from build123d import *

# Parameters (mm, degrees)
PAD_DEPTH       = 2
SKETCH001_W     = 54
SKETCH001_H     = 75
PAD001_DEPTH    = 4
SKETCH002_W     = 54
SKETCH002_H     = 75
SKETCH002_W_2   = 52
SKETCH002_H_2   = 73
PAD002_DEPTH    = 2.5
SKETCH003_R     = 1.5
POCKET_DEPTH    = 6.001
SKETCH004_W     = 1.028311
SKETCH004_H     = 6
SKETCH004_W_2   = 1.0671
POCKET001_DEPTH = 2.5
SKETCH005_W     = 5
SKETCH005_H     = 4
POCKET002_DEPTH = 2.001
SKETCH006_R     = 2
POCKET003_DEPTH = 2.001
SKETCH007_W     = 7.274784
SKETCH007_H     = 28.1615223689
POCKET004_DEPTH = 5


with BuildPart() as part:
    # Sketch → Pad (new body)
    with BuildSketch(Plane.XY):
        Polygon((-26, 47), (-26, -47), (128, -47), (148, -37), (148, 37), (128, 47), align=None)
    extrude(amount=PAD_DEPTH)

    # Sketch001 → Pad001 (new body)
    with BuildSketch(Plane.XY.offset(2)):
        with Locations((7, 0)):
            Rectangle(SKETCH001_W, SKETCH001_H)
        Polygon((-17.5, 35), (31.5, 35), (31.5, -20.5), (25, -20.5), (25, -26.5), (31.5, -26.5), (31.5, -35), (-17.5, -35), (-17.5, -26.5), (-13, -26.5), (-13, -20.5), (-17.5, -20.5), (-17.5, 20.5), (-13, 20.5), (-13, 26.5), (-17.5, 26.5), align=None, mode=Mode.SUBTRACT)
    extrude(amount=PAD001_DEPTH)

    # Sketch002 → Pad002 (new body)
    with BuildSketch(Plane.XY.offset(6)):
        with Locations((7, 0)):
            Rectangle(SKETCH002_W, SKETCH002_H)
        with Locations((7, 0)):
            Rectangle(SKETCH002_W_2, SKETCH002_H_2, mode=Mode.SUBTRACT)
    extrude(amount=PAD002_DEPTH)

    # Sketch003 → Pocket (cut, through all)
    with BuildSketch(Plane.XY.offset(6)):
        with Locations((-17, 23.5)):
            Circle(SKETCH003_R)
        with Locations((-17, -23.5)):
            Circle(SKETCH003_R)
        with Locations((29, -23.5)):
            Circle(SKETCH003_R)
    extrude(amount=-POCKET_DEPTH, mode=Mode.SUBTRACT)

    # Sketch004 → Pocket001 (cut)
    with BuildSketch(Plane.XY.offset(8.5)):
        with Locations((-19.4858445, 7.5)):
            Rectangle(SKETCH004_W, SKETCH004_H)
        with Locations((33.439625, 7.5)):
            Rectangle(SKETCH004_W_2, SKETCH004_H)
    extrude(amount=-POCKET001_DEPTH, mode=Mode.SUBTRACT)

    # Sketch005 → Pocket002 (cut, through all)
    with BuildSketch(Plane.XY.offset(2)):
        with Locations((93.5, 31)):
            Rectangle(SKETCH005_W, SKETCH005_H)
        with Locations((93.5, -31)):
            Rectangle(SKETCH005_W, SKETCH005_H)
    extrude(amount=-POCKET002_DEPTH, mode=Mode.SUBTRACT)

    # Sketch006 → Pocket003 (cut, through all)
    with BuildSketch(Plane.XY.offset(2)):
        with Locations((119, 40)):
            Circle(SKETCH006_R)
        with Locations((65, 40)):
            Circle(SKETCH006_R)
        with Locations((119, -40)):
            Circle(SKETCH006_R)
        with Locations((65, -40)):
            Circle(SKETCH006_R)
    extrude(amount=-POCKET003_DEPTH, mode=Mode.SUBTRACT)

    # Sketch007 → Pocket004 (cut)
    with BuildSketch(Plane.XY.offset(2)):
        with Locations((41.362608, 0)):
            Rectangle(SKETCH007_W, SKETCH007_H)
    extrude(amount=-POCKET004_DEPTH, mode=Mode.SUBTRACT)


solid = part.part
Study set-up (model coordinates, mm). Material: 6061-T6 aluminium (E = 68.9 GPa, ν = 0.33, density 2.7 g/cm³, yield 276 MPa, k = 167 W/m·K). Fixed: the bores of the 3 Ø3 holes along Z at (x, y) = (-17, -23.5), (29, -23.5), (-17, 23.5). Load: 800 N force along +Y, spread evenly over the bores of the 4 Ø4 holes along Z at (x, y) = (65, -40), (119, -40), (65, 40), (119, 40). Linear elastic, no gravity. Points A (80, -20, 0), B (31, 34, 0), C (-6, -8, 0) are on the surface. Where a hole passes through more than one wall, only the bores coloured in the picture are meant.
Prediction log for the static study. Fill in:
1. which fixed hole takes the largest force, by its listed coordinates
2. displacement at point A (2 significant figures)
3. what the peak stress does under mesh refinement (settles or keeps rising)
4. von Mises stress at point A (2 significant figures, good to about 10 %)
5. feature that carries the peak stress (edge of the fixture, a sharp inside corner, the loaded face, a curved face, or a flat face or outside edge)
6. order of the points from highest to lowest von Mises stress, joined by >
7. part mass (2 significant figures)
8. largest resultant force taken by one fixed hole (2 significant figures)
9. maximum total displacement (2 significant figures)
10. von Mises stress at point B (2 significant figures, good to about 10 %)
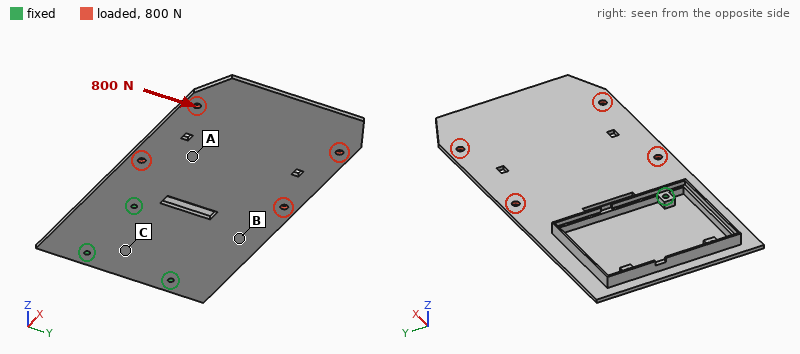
(29, -23.5)
36 µm
keeps rising
6.1 MPa
edge of the fixture
B > A > C
95 g
1.2 kN
80 µm
13 MPa
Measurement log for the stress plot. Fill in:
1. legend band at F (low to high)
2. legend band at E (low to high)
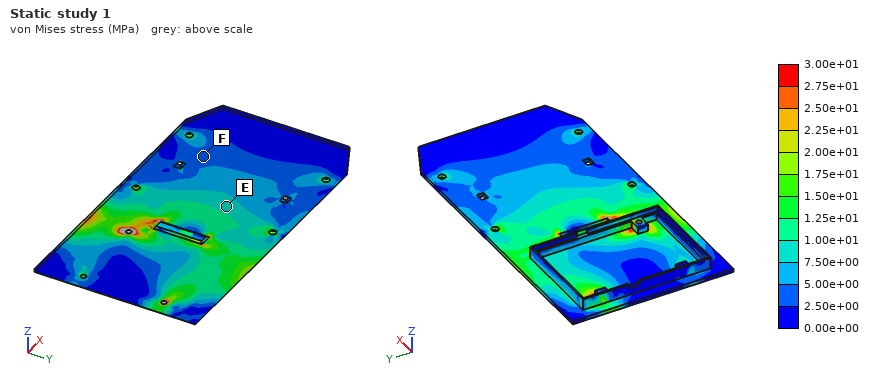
2.50e+00 to 5.00e+00 MPa
7.50e+00 to 1.00e+01 MPa
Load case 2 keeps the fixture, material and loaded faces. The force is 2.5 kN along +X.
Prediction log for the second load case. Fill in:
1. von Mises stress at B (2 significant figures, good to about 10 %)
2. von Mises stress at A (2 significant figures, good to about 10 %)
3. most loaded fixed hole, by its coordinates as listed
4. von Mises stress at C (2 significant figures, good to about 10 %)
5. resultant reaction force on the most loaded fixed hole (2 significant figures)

18 MPa
9.0 MPa
(29, -23.5)
5.3 MPa
1.2 kN
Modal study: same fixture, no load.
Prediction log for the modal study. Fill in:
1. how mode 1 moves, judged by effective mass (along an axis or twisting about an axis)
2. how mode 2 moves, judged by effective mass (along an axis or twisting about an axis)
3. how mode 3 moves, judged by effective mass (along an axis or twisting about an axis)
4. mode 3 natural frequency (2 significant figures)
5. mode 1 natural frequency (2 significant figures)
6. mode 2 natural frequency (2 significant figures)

along Z
twisting about X
along Z
650 Hz
110 Hz
330 Hz
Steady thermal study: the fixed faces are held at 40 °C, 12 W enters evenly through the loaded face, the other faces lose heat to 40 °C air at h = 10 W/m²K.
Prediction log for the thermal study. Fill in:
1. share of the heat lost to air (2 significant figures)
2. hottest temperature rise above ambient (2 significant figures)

35 %
27 K
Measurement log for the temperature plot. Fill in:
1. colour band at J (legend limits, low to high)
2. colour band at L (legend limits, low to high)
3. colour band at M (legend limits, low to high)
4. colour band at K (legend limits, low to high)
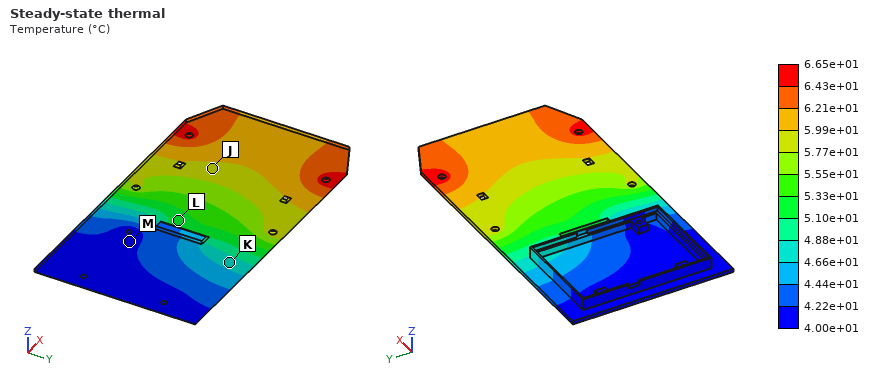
5.77e+01 to 5.99e+01 °C
5.10e+01 to 5.33e+01 °C
4.00e+01 to 4.22e+01 °C
4.66e+01 to 4.88e+01 °C
